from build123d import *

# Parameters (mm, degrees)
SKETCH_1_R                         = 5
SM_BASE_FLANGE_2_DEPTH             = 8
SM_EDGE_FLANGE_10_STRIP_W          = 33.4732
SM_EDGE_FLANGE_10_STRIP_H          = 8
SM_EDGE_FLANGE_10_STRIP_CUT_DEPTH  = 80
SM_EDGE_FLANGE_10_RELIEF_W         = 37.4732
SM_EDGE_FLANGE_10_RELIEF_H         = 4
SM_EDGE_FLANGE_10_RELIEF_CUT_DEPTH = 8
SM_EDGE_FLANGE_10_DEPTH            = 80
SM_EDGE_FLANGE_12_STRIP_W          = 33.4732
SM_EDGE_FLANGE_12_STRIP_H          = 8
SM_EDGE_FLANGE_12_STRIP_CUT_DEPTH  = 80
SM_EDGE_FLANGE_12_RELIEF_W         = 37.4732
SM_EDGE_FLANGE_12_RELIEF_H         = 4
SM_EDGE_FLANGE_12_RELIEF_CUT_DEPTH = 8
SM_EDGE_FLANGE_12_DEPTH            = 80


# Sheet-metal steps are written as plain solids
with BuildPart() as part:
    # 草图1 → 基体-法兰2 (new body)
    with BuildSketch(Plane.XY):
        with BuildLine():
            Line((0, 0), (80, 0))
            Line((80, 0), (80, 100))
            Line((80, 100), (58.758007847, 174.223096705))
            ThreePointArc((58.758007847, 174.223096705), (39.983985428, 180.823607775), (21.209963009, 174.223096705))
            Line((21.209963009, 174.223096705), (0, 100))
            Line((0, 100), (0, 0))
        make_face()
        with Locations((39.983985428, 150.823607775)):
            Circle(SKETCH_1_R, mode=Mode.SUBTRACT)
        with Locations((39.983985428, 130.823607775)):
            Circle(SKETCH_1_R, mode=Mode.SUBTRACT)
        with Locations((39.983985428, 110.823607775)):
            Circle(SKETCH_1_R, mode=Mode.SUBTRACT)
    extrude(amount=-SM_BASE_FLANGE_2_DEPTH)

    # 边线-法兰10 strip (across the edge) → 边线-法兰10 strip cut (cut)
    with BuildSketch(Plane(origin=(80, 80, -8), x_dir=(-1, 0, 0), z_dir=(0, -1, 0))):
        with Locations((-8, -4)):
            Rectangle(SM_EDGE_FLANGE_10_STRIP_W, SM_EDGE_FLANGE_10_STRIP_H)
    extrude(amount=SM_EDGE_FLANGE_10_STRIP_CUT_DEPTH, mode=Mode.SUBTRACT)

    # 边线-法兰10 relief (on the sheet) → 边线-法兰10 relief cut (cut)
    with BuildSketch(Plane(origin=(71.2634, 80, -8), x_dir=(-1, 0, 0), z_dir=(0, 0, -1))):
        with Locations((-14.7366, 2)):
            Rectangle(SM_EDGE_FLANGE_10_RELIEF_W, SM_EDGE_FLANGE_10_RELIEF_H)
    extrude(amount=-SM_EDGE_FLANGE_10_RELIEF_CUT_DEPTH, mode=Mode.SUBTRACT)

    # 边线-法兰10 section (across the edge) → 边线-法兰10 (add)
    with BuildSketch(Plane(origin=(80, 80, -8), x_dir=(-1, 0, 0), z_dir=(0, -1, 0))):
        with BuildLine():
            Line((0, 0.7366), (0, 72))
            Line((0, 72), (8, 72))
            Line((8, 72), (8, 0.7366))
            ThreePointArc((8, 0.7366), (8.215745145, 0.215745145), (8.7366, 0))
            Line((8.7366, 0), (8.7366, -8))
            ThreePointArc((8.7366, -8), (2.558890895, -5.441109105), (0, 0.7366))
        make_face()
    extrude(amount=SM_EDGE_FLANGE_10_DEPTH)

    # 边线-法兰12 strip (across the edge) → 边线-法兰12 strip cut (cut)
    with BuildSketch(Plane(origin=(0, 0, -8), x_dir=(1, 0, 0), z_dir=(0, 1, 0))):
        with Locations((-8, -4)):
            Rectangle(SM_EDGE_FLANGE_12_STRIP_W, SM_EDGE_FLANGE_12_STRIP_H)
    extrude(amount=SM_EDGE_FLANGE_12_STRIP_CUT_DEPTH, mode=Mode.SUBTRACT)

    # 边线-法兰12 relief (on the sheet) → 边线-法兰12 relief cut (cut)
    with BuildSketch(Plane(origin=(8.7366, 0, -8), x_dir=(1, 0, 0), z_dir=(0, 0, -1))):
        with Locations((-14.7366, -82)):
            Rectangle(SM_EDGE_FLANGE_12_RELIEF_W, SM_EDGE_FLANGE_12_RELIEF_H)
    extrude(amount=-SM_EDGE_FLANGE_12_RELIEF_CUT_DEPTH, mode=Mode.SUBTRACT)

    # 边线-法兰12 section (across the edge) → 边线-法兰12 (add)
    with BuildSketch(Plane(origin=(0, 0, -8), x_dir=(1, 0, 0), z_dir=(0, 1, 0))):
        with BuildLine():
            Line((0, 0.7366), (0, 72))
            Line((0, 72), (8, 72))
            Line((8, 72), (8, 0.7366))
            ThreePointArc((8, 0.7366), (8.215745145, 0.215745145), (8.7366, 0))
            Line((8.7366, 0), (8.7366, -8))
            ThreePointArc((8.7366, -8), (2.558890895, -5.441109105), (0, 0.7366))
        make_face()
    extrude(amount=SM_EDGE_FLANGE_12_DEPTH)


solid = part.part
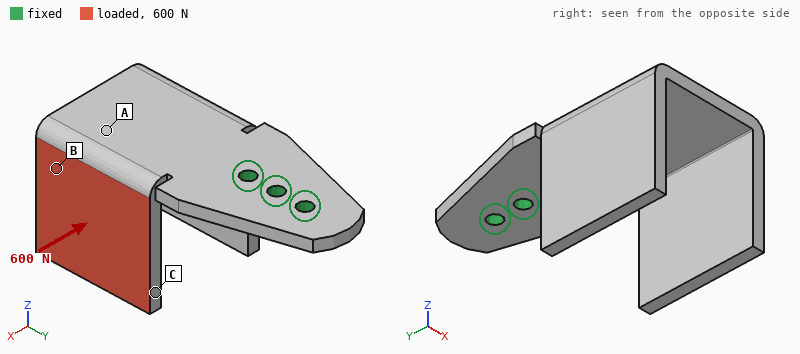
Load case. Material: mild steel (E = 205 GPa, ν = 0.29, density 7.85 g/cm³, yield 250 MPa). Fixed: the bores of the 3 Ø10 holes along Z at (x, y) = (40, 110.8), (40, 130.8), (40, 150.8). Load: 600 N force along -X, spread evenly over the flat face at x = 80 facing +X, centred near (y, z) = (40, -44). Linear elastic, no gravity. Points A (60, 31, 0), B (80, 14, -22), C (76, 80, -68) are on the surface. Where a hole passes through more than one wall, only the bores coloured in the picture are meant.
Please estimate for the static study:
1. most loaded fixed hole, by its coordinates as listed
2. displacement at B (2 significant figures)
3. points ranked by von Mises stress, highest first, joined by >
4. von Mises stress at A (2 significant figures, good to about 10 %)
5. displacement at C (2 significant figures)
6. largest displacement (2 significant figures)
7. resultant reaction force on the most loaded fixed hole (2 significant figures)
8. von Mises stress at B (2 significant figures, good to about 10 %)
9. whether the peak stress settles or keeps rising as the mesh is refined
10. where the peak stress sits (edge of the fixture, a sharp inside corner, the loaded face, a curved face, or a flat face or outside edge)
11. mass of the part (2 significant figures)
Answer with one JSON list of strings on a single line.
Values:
["(40, 110.8)", "0.093 mm", "A > B > C", "21 MPa", "0.18 mm", "0.24 mm", "1.5 kN", "13 MPa", "keeps rising", "a sharp inside corner", "1.5 kg"]
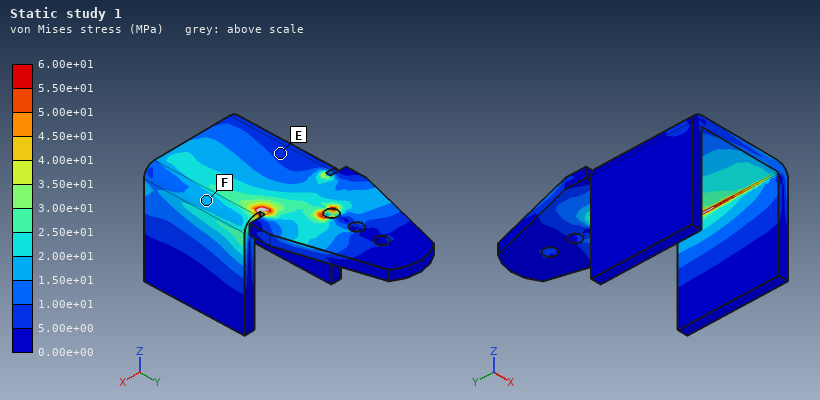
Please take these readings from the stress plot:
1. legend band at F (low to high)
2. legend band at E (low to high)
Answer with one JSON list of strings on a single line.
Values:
["1.50e+01 to 2.00e+01 MPa", "5.00e+00 to 1.00e+01 MPa"]
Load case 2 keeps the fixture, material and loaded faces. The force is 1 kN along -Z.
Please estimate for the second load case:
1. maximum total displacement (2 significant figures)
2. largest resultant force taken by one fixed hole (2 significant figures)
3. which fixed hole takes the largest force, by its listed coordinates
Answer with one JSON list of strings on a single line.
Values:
["0.63 mm", "2.2 kN", "(40, 110.8)"]
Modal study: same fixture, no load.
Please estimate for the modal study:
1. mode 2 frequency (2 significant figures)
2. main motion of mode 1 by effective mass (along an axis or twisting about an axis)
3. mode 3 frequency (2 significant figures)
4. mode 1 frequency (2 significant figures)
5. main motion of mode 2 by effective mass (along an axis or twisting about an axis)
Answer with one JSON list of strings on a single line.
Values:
["370 Hz", "along Z", "710 Hz", "260 Hz", "along X"]
